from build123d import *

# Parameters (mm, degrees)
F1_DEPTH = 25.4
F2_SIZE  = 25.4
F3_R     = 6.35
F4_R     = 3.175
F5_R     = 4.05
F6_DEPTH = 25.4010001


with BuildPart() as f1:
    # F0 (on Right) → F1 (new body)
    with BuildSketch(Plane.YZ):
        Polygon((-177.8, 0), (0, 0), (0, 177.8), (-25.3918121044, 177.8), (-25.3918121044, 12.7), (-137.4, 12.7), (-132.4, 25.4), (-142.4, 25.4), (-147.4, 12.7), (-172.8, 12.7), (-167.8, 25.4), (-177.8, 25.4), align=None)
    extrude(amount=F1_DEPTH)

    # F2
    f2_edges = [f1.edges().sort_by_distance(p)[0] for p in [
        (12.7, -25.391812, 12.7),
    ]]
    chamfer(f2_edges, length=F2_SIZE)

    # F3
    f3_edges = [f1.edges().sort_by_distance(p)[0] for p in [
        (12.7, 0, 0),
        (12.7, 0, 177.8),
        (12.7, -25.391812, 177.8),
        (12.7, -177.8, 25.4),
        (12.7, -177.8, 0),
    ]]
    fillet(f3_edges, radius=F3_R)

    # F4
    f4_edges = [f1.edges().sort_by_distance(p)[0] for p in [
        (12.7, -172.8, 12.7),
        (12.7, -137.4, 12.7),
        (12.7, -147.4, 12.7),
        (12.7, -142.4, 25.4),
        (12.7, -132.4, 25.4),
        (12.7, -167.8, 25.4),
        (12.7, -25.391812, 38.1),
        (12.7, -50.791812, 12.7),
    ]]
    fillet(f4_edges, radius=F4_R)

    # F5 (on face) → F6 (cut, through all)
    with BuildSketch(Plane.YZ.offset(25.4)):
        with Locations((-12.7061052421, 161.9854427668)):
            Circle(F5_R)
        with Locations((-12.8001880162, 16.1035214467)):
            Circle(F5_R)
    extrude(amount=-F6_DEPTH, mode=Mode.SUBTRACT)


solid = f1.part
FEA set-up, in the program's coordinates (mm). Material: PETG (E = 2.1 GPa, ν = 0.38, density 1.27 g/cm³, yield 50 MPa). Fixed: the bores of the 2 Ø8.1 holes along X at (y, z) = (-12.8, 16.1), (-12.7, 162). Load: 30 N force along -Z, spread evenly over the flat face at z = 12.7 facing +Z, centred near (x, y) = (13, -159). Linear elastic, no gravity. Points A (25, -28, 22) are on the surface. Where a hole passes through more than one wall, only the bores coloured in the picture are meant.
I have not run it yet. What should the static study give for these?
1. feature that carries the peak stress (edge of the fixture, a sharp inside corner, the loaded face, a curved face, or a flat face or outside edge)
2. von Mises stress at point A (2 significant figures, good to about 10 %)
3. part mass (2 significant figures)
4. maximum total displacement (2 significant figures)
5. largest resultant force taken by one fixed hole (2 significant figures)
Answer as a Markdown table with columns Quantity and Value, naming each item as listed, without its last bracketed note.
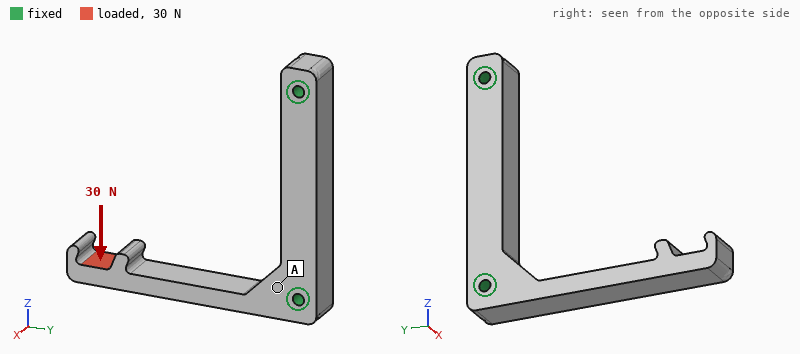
| Quantity | Value |
|---|---|
| feature that carries the peak stress | a curved face |
| von Mises stress at point A | 0.56 MPa |
| part mass | 220 g |
| maximum total displacement | 2.3 mm |
| largest resultant force taken by one fixed hole | 22 N |
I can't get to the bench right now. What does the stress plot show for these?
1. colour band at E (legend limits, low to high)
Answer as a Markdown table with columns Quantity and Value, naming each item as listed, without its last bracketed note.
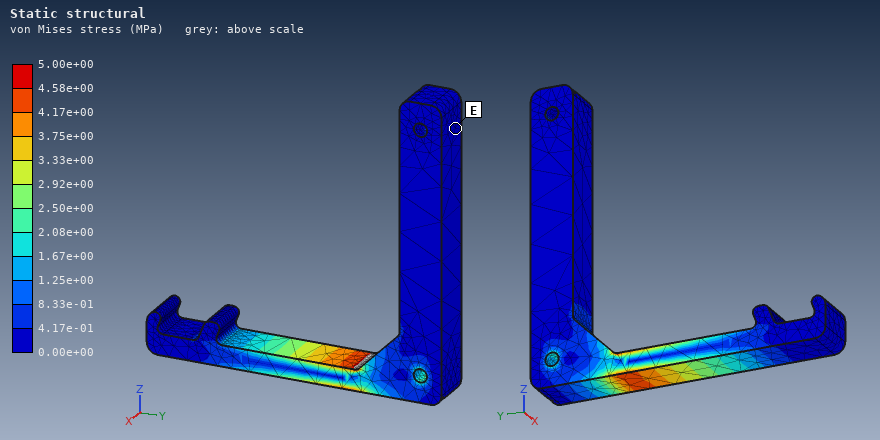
| Quantity | Value |
|---|---|
| colour band at E | 0.00e+00 to 4.17e-01 MPa |
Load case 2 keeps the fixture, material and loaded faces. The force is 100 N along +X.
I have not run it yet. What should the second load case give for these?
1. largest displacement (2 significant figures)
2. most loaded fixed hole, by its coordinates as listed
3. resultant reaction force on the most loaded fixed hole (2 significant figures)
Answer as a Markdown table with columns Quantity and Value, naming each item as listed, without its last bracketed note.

| Quantity | Value |
|---|---|
| largest displacement | 2.8 mm |
| most loaded fixed hole, by its coordinates as listed | (-12.8, 16.1) |
| resultant reaction force on the most loaded fixed hole | 110 N |
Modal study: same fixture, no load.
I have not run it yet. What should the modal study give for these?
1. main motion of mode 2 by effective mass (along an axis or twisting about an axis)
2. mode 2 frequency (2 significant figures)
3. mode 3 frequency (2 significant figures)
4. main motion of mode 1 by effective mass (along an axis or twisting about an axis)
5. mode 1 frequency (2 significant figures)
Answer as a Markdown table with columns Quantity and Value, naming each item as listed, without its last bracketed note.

| Quantity | Value |
|---|---|
| main motion of mode 2 by effective mass | along X |
| mode 2 frequency | 200 Hz |
| mode 3 frequency | 700 Hz |
| main motion of mode 1 by effective mass | along Z |
| mode 1 frequency | 120 Hz |
